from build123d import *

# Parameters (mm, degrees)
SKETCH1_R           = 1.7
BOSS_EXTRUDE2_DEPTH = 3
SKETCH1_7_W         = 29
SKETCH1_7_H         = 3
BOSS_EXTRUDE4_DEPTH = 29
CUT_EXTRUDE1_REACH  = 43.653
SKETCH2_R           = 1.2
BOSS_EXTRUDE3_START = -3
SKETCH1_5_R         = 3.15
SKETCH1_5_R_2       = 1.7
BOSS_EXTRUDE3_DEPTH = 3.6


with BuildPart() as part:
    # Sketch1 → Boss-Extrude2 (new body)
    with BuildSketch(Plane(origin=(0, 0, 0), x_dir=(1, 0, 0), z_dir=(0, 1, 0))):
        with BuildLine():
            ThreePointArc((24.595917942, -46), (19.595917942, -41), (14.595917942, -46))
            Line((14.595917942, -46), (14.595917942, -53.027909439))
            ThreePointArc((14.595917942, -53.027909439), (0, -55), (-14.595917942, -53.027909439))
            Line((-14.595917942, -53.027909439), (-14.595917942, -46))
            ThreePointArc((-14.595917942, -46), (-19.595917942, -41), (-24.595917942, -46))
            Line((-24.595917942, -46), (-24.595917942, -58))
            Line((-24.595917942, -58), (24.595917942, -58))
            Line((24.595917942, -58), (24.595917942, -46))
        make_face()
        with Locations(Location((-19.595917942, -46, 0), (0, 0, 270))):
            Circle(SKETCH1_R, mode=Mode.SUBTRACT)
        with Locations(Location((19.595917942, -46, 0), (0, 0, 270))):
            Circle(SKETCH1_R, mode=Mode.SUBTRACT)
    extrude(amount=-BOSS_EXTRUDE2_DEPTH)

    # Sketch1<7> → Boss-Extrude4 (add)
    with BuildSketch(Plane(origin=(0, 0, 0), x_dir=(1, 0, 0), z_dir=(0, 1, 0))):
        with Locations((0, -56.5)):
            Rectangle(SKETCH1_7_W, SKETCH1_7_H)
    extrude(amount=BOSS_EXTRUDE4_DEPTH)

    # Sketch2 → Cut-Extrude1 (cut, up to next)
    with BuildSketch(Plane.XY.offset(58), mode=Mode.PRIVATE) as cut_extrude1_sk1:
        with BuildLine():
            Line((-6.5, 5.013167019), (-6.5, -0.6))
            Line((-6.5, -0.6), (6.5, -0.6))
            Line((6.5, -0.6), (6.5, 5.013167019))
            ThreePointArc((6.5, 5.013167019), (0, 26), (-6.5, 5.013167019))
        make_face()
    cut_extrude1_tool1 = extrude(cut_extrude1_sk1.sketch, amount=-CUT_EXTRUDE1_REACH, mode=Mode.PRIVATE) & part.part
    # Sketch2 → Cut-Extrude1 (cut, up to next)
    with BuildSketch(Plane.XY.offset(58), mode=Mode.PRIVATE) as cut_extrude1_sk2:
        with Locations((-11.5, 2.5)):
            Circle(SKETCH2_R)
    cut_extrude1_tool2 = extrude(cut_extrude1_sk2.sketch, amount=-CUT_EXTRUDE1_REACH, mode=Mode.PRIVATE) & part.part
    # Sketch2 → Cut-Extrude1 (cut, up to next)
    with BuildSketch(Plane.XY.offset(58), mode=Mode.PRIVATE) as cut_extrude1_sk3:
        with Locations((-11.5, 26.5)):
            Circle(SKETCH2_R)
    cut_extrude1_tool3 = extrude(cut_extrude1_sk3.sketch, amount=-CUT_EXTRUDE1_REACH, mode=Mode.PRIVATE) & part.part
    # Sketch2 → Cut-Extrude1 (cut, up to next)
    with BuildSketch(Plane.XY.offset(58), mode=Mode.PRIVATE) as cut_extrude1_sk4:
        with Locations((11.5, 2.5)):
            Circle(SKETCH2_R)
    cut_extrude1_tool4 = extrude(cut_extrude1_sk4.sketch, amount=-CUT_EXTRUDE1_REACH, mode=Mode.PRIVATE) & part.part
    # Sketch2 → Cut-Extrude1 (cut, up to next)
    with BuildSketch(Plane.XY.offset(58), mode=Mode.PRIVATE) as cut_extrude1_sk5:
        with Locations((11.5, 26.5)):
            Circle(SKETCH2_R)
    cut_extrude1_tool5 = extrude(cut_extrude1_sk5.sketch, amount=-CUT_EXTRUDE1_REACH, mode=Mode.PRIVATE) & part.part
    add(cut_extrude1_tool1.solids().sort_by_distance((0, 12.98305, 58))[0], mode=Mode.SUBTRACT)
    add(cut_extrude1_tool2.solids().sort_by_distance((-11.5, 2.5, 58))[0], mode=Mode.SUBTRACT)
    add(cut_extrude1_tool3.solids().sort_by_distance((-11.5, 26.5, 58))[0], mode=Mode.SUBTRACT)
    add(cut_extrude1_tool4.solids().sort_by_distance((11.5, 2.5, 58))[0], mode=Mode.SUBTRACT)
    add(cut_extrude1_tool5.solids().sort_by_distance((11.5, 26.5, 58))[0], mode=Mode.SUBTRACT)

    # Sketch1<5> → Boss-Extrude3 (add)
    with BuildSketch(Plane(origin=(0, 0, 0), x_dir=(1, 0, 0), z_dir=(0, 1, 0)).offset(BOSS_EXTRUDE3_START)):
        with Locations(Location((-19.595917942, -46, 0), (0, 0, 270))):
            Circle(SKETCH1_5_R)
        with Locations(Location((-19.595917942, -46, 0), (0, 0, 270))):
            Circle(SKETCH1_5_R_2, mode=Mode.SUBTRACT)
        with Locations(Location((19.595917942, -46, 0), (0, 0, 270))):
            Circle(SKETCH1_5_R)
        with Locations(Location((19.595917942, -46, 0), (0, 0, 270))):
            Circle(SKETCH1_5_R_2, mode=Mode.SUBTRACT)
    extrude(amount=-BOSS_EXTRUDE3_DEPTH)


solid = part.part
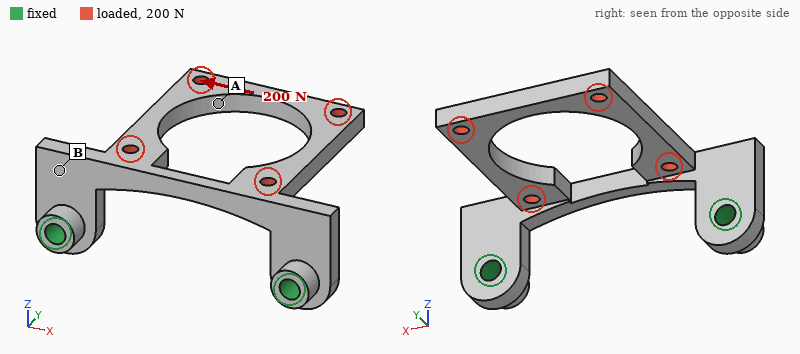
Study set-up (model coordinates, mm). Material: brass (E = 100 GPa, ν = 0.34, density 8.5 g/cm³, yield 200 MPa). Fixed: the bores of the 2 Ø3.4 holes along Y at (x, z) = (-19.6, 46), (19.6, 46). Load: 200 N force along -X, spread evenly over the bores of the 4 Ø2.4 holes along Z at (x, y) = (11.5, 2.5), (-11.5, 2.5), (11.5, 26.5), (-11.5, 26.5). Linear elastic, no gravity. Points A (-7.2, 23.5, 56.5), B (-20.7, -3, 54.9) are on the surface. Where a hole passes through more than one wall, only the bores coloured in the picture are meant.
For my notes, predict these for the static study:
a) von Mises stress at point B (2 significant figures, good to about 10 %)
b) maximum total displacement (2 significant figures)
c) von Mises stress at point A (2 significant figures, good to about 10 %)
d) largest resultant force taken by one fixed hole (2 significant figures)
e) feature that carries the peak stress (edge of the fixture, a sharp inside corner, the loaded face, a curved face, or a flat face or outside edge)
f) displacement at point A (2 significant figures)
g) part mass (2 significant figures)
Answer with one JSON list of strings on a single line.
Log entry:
["11 MPa", "66 µm", "35 MPa", "130 N", "a flat face or outside edge", "57 µm", "21 g"]
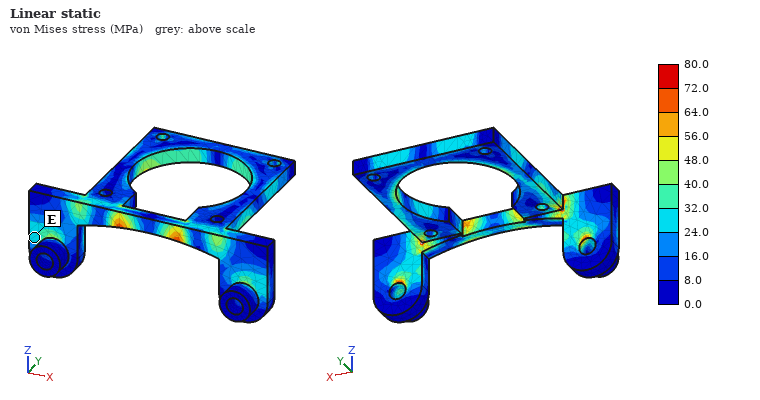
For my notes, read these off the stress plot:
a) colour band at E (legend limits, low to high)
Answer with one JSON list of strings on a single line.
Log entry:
["24.0 to 32.0 MPa"]
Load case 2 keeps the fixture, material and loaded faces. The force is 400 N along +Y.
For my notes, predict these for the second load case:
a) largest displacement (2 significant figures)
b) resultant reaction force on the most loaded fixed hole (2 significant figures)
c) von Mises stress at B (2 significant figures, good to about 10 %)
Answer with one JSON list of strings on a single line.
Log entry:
["0.15 mm", "200 N", "46 MPa"]
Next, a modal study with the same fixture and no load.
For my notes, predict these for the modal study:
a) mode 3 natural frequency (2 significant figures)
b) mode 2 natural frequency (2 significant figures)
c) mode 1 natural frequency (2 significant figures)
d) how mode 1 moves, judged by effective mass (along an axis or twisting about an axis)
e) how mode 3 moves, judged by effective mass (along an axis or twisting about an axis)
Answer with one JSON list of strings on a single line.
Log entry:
["3200 Hz", "2500 Hz", "970 Hz", "along Z", "along X"]
